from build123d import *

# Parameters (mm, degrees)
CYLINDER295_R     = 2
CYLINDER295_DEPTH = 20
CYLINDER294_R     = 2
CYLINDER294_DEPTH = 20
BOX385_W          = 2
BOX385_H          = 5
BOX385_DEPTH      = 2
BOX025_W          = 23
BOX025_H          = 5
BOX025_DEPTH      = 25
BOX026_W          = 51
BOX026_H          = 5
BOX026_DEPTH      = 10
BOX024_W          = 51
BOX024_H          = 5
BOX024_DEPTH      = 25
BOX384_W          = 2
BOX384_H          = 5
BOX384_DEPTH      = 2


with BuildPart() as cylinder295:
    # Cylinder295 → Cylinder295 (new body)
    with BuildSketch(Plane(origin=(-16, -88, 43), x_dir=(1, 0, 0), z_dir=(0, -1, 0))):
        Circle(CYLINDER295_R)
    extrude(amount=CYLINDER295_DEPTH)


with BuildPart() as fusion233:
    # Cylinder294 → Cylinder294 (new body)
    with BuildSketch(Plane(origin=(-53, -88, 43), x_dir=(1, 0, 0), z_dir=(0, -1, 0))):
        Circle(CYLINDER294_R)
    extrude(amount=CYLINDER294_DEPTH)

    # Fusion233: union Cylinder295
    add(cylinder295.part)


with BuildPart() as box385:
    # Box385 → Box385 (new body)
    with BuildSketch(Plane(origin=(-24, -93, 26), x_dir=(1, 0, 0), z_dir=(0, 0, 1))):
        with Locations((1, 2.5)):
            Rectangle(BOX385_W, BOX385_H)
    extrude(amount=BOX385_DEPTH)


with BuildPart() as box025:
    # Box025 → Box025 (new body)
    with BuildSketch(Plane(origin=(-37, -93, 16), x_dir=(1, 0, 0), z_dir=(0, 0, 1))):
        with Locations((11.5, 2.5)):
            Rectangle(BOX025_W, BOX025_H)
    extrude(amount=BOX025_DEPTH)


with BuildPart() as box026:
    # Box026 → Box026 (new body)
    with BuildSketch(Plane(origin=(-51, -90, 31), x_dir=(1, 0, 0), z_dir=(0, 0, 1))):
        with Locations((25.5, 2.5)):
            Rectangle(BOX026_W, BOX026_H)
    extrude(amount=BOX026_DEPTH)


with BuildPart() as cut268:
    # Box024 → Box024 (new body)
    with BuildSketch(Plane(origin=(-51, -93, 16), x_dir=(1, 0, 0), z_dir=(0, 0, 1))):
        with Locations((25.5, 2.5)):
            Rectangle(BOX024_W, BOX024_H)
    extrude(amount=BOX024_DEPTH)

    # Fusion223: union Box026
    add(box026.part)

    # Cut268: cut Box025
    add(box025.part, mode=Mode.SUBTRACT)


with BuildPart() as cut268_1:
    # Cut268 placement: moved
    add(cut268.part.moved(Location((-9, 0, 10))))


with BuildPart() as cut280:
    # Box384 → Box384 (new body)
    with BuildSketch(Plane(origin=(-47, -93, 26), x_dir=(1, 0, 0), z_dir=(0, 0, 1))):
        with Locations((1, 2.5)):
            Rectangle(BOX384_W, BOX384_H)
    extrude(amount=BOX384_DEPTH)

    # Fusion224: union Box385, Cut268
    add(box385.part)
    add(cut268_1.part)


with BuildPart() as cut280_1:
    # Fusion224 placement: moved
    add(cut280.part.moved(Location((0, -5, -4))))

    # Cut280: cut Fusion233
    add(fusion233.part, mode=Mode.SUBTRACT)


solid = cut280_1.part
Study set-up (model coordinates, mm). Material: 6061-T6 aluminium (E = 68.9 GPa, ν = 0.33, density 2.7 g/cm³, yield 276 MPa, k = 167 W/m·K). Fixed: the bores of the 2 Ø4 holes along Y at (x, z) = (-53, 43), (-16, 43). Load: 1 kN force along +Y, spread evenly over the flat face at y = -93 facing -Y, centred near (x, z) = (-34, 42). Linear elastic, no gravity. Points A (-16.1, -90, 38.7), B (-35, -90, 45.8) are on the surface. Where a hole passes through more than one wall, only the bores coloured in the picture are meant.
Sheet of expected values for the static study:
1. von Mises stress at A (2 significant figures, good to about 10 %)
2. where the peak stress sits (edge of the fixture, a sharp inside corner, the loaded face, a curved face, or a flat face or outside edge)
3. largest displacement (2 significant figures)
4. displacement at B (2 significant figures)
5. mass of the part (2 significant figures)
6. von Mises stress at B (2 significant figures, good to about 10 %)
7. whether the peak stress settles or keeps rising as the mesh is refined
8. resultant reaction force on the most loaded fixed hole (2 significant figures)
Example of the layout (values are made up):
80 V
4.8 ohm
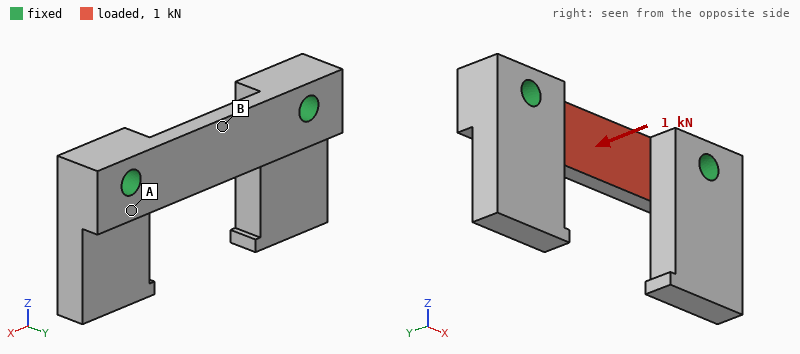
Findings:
13 MPa
a sharp inside corner
43 µm
41 µm
13 g
89 MPa
keeps rising
550 N
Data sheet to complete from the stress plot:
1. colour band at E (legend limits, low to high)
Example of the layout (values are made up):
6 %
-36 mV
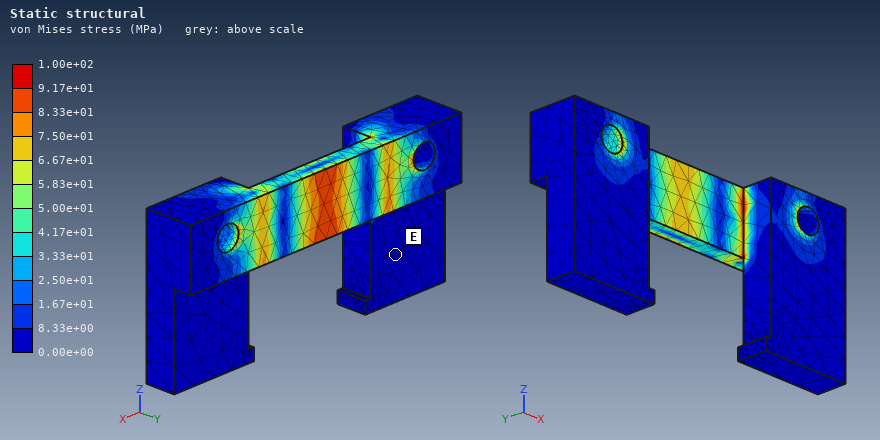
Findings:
0.00e+00 to 8.33e+00 MPa
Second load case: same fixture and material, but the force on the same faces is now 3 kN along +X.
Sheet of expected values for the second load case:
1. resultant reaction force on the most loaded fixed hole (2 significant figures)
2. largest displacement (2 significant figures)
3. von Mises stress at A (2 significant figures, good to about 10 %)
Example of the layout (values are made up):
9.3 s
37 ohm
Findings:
1.5 kN
10 µm
23 MPa
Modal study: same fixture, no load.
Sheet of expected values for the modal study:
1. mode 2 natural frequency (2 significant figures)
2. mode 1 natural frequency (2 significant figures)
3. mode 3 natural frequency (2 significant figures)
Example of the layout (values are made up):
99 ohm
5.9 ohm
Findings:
12 kHz
12 kHz
16 kHz
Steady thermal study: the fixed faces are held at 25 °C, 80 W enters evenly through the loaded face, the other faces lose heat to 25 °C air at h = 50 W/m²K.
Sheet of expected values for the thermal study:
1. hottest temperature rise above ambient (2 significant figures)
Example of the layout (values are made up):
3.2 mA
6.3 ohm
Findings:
73 K
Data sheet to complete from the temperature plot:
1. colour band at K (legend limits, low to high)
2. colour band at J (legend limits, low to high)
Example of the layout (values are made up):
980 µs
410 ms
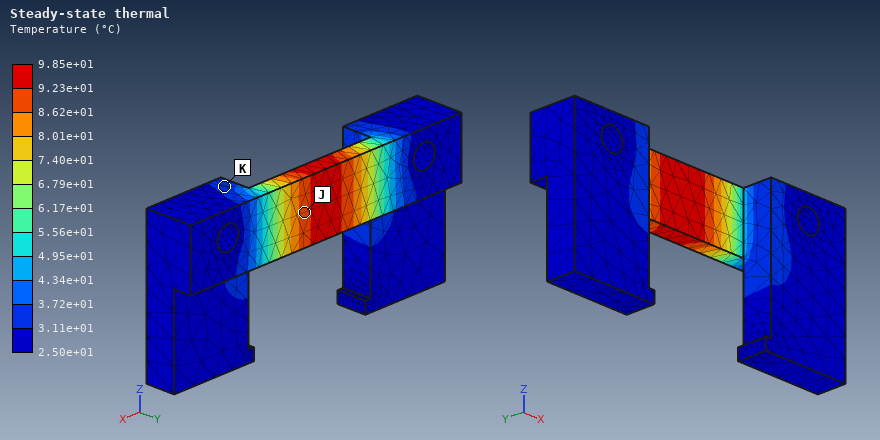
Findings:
3.11e+01 to 3.72e+01 °C
8.62e+01 to 9.23e+01 °C
